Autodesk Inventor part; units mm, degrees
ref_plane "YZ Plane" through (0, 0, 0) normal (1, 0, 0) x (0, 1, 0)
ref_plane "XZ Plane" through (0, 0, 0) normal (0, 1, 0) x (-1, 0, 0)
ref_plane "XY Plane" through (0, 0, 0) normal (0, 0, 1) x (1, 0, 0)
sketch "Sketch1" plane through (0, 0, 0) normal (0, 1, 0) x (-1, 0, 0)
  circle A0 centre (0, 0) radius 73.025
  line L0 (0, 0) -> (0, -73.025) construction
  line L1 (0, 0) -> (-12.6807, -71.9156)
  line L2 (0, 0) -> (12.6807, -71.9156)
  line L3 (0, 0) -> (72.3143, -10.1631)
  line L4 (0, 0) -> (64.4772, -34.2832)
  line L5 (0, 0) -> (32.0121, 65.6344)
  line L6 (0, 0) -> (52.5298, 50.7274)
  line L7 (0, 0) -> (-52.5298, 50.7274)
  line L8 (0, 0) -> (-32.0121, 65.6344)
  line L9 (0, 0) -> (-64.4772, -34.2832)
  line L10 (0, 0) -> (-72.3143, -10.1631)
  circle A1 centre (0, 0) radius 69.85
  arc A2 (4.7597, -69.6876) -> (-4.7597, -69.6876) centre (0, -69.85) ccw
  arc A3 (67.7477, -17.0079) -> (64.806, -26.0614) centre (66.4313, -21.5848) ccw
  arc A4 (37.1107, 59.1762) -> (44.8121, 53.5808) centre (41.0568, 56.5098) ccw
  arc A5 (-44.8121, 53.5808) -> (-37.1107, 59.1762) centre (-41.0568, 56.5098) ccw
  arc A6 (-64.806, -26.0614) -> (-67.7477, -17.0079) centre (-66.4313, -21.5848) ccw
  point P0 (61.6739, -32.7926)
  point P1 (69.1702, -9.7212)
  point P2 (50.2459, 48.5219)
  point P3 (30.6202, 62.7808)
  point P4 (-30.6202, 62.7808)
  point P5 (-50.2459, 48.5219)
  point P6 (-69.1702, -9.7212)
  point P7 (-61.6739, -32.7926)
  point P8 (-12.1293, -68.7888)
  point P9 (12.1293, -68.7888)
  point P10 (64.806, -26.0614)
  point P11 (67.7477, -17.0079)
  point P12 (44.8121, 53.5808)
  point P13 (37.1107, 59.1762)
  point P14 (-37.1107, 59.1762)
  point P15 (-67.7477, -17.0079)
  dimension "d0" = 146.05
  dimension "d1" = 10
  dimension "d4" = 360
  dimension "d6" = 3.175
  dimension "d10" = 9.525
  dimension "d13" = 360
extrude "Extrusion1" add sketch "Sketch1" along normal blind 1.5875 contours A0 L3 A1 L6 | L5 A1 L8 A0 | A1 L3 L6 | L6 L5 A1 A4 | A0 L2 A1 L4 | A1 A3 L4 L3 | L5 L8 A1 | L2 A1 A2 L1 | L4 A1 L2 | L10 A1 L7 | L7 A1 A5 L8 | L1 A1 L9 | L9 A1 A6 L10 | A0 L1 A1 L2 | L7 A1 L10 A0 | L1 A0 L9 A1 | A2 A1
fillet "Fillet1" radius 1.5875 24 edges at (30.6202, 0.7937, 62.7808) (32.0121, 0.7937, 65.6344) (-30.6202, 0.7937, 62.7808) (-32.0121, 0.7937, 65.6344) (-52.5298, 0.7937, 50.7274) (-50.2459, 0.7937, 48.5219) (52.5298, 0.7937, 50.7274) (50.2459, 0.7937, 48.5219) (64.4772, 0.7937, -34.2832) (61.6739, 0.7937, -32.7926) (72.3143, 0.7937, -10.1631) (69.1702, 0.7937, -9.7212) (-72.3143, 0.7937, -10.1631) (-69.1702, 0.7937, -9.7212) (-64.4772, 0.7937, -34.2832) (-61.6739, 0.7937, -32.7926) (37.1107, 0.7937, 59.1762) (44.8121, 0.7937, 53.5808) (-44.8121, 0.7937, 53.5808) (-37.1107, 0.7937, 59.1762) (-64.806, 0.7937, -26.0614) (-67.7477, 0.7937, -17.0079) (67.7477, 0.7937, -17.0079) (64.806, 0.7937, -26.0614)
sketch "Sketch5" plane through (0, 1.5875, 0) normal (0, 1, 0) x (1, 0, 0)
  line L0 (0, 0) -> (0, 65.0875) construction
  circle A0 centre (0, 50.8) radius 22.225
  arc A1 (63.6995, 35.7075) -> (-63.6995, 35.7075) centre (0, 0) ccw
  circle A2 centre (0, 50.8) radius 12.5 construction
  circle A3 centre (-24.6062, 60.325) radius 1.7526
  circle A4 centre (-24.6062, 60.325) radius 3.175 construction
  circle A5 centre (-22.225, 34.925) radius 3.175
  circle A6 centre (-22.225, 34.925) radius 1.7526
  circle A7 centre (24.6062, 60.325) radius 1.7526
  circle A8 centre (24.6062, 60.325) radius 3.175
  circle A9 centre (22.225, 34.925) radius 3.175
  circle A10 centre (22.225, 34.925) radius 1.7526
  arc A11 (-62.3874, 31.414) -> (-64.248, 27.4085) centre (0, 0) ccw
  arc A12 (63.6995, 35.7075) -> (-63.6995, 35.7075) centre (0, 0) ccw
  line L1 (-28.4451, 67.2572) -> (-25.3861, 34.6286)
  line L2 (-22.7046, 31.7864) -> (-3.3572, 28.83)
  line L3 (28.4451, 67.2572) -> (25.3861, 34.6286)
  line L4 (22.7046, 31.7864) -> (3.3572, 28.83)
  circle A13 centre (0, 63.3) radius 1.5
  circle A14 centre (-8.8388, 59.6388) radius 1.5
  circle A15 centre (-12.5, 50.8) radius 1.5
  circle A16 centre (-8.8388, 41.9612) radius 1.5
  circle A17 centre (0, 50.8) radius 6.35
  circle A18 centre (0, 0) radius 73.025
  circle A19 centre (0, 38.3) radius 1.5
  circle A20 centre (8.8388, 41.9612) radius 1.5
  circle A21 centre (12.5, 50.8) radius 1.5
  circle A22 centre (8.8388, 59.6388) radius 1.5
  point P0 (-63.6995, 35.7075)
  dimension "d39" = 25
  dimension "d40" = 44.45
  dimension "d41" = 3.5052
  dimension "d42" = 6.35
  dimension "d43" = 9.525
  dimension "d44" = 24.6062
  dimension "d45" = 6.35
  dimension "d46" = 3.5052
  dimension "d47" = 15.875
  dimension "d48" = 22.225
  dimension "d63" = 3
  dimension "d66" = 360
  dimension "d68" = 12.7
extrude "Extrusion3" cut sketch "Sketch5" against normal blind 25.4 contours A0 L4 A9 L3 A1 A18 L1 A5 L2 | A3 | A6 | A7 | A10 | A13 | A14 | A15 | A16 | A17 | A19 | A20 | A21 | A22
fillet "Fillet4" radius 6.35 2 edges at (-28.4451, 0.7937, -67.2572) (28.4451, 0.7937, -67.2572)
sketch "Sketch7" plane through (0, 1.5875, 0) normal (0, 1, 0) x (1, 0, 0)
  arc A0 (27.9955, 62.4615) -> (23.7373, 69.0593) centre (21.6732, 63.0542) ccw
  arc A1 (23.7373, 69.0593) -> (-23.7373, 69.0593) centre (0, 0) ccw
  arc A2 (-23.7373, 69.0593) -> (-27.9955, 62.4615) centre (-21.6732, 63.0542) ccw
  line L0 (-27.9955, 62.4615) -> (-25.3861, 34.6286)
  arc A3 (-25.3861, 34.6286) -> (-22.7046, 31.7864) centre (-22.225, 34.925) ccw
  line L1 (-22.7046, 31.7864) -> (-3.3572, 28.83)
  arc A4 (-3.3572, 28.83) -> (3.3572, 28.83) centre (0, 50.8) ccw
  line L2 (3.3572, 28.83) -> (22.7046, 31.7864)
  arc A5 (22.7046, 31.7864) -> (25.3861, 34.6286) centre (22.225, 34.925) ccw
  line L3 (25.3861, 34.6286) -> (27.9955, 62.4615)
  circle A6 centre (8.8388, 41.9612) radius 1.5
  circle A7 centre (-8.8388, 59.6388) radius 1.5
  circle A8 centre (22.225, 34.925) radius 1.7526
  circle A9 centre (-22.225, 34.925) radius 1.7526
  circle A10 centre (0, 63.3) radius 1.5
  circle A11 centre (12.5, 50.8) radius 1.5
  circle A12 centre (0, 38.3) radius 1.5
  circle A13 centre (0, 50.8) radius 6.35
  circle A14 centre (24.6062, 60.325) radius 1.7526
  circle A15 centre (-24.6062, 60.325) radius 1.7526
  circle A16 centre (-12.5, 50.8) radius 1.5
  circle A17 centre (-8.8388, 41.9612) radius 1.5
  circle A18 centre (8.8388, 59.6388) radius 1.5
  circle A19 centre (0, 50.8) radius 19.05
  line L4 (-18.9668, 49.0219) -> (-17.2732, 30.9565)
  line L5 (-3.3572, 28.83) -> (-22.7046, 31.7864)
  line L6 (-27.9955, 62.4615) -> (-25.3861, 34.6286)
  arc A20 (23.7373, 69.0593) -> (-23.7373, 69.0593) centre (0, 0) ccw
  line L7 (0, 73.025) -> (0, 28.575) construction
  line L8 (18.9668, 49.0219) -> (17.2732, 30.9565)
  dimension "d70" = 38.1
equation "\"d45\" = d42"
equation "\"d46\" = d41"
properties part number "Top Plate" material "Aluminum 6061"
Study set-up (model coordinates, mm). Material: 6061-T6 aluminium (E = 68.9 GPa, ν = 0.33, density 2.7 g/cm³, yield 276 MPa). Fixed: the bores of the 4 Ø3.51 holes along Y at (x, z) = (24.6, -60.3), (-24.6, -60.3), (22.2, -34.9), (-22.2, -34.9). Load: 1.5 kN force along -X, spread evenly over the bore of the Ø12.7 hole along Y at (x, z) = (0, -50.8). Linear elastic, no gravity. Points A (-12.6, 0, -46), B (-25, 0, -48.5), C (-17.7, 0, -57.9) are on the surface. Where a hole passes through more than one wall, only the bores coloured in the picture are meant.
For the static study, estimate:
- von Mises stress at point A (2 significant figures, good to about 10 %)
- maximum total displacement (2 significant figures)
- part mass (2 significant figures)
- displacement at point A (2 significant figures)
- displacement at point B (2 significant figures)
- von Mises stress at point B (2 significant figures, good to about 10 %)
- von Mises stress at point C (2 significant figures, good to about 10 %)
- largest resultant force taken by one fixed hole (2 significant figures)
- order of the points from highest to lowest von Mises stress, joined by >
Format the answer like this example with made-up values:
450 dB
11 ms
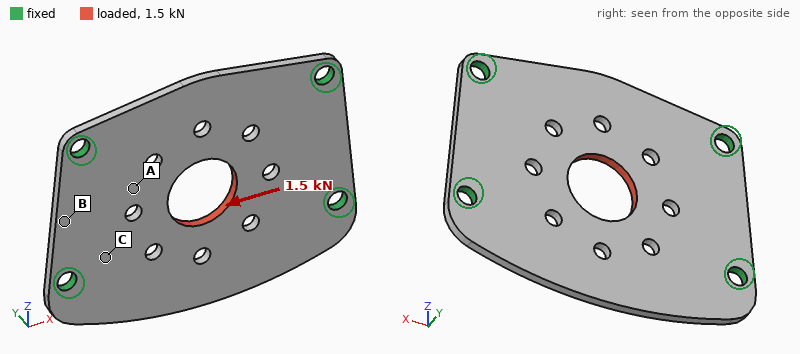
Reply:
17 MPa
8.1 µm
8.4 g
5.0 µm
3.8 µm
6.8 MPa
28 MPa
440 N
C > A > B
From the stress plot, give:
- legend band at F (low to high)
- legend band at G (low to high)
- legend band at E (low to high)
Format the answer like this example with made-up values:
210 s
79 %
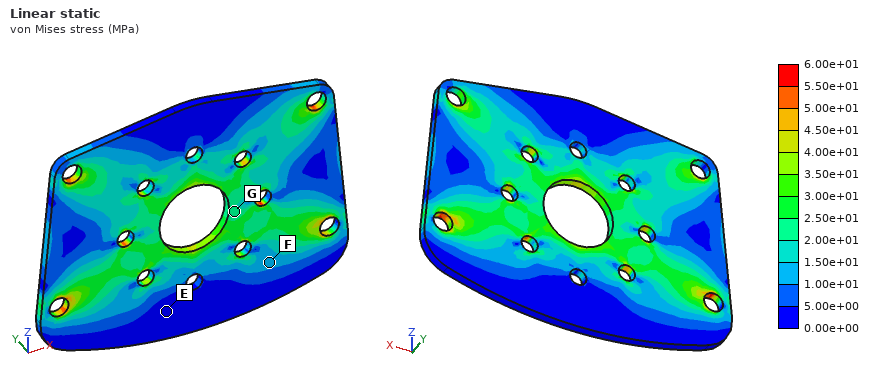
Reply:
1.00e+01 to 1.50e+01 MPa
2.00e+01 to 2.50e+01 MPa
0.00e+00 to 5.00e+00 MPa
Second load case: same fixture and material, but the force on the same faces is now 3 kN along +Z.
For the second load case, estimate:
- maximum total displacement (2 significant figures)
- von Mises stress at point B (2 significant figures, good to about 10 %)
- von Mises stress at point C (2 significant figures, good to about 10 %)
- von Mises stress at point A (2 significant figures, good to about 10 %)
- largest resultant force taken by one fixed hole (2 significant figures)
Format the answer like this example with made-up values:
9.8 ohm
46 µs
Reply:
31 µm
12 MPa
46 MPa
62 MPa
910 N
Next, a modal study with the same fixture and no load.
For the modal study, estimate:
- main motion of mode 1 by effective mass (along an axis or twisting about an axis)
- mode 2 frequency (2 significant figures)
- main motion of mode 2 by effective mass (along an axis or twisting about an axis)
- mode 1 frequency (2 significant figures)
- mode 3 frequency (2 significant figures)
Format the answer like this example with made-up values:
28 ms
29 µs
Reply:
along Y
4400 Hz
along Y
3300 Hz
6800 Hz
